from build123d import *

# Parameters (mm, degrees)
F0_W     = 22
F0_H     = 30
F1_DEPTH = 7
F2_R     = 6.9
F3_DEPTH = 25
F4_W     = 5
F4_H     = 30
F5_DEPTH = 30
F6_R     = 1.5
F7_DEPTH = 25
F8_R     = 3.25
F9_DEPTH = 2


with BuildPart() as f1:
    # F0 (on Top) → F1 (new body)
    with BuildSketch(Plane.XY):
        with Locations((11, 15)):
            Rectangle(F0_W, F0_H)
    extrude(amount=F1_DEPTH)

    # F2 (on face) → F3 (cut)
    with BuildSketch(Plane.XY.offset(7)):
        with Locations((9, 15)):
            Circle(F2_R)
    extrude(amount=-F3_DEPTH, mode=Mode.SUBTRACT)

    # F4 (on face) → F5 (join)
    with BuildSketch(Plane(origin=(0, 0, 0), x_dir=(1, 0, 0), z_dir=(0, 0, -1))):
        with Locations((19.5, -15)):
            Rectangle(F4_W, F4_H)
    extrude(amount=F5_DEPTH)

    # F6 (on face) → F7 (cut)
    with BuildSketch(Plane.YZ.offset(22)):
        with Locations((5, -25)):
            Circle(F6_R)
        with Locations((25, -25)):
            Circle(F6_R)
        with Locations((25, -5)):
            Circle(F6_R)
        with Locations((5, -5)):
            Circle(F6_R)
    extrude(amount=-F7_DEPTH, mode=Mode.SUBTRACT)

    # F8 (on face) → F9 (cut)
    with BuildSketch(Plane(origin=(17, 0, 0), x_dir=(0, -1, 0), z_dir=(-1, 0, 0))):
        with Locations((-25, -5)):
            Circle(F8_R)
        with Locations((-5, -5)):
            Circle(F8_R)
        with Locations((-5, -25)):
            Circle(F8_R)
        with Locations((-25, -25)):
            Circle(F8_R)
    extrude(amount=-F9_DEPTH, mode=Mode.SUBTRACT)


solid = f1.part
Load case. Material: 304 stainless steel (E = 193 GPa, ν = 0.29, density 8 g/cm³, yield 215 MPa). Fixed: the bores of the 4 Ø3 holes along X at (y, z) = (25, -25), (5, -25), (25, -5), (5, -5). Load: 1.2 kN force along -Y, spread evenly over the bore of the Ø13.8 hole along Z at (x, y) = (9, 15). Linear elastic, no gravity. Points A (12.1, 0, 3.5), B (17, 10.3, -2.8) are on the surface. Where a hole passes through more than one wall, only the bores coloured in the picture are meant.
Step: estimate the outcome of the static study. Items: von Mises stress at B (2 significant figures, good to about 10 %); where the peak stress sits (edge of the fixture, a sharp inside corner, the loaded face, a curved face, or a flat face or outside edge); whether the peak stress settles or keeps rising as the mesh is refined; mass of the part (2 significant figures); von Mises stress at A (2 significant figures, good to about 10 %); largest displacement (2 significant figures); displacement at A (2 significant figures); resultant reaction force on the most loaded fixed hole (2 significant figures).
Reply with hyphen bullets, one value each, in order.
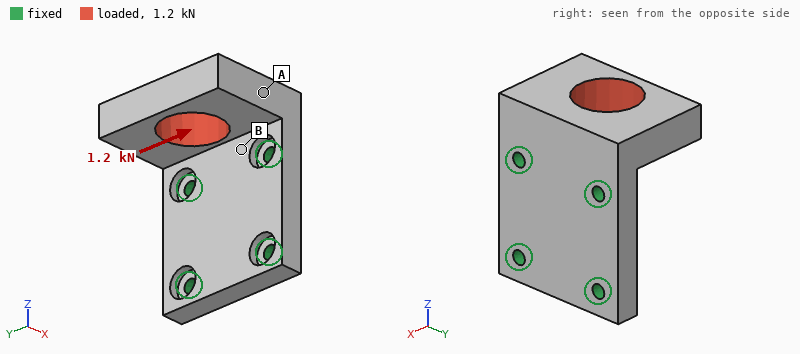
- 36 MPa
- edge of the fixture
- keeps rising
- 62 g
- 17 MPa
- 16 µm
- 8.7 µm
- 980 N
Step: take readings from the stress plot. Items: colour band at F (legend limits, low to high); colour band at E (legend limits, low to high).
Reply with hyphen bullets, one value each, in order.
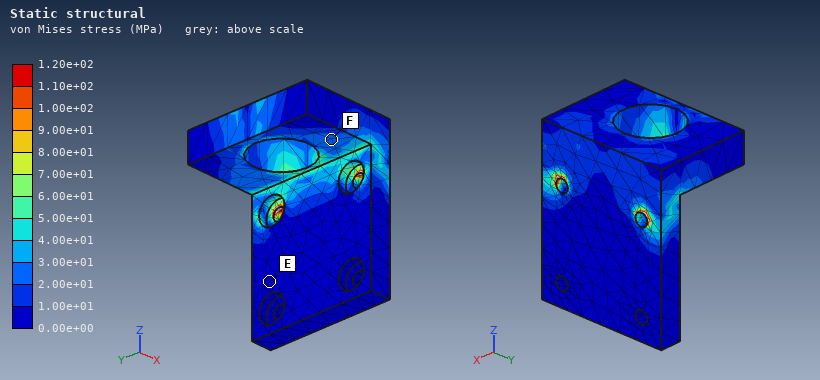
- 2.00e+01 to 3.00e+01 MPa
- 0.00e+00 to 1.00e+01 MPa
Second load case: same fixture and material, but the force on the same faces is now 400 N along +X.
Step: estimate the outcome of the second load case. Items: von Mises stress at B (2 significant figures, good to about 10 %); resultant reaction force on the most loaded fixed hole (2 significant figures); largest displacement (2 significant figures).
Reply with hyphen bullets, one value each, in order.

- 20 MPa
- 260 N
- 10 µm
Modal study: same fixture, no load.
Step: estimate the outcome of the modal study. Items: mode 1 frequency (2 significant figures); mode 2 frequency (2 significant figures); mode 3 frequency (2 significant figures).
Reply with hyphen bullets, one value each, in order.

- 5200 Hz
- 9700 Hz
- 15 kHz
